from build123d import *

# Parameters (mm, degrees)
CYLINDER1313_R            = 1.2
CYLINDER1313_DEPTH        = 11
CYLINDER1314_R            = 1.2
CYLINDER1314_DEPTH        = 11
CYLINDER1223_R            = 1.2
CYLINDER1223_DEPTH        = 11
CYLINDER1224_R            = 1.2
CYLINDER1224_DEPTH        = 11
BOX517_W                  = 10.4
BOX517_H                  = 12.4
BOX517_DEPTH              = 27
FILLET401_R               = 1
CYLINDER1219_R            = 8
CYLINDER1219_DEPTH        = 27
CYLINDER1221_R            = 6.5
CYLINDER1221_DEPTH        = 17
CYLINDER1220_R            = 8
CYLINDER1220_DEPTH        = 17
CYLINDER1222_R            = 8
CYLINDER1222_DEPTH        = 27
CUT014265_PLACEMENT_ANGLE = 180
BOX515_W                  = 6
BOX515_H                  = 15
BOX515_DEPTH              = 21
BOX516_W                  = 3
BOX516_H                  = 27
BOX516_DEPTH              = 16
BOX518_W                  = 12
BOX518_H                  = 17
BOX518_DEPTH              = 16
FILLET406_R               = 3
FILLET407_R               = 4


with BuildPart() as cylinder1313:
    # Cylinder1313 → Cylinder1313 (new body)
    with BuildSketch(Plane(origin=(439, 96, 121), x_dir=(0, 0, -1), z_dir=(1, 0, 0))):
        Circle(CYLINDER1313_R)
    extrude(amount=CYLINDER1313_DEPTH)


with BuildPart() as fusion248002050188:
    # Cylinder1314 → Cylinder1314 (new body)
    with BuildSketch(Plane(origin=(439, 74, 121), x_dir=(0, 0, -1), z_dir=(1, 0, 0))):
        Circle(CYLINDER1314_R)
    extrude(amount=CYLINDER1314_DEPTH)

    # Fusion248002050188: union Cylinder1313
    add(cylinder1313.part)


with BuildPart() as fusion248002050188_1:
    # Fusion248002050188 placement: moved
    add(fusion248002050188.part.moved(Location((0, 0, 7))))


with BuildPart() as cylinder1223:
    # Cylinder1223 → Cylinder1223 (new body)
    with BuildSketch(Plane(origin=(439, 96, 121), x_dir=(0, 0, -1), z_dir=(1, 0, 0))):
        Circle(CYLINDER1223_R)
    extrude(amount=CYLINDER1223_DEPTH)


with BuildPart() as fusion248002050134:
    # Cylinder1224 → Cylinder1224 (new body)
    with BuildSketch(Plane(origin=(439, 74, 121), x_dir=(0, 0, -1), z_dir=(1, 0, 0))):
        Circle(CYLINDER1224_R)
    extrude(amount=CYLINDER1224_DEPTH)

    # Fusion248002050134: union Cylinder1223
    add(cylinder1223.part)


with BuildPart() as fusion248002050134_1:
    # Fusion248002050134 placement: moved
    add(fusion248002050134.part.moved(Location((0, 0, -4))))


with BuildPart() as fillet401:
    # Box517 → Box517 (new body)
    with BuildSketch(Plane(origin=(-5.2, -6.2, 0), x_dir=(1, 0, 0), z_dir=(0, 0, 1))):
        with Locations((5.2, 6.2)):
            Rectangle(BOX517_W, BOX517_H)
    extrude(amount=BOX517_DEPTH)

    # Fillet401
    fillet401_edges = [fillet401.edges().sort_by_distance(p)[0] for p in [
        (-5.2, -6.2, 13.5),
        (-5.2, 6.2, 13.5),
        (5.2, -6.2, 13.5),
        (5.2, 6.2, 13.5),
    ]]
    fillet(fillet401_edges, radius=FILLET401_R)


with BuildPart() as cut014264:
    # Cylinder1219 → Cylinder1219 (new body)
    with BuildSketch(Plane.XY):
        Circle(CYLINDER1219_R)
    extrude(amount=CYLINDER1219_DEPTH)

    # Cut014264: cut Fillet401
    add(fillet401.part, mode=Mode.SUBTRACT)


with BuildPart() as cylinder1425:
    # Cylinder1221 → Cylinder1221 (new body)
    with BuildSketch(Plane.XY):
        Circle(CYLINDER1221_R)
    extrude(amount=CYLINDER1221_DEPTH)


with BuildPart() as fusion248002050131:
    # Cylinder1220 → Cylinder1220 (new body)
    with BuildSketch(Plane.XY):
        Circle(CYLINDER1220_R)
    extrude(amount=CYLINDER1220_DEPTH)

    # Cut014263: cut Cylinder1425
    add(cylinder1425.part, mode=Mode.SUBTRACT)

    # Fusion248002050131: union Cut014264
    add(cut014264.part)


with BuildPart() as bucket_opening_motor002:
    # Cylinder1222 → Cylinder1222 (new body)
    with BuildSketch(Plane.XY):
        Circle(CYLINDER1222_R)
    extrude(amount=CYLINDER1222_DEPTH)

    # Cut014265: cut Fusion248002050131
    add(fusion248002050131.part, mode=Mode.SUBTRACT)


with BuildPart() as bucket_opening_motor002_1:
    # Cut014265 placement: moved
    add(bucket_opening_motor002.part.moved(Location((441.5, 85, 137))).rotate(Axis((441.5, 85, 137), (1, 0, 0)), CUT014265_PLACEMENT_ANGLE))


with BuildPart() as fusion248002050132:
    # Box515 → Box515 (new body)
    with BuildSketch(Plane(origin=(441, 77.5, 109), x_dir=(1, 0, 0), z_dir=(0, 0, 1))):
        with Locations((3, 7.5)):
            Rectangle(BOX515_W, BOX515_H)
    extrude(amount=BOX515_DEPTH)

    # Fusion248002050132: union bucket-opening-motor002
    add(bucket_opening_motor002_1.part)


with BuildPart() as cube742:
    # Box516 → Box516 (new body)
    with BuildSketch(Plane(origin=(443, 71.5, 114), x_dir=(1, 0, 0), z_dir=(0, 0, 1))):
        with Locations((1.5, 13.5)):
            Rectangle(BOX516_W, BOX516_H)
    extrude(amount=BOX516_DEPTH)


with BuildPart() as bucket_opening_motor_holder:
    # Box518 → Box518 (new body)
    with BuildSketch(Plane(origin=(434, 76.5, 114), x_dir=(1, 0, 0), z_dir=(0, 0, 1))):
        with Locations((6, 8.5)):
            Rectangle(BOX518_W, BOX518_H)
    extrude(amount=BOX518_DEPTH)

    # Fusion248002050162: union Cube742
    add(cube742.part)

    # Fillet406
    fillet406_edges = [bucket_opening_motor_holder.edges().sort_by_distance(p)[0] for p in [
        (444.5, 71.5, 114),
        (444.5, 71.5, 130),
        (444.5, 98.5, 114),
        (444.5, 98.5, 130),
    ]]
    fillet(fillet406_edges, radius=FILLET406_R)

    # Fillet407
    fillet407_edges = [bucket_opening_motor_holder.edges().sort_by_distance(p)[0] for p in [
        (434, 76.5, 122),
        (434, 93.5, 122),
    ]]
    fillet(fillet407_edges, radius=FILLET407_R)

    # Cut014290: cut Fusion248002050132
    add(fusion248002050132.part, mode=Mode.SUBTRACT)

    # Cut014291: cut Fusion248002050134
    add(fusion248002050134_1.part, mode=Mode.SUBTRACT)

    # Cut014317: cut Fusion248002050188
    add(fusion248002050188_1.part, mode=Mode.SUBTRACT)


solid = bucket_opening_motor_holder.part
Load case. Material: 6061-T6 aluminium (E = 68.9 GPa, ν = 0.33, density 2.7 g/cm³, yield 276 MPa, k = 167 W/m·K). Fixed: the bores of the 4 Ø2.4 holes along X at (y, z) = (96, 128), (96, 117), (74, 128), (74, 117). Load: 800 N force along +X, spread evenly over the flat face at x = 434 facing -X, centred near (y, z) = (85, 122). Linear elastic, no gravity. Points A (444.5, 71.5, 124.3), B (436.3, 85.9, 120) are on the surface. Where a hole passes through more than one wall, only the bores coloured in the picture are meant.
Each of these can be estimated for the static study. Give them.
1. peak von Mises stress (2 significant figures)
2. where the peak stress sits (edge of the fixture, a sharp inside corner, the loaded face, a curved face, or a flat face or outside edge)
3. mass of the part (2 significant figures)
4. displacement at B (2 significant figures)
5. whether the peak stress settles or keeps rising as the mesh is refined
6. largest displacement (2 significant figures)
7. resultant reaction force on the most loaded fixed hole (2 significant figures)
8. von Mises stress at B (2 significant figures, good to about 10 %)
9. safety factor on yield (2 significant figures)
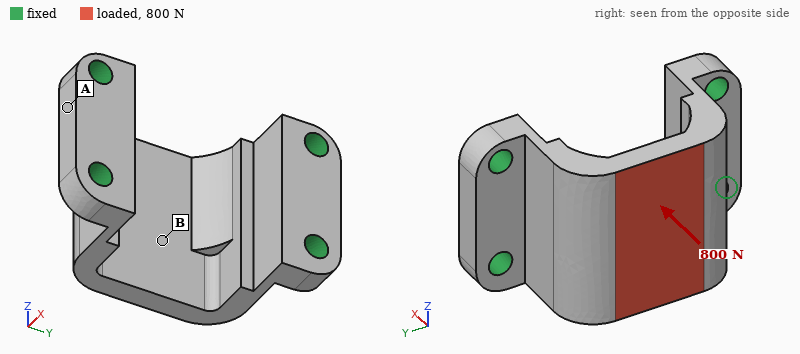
100 MPa
a curved face
4.0 g
14 µm
settles
19 µm
240 N
44 MPa
2.7
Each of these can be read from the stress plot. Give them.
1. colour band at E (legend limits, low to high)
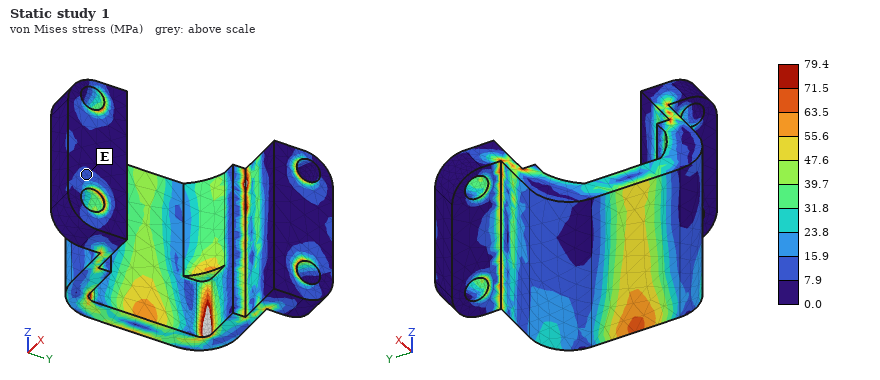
7.9 to 15.9 MPa
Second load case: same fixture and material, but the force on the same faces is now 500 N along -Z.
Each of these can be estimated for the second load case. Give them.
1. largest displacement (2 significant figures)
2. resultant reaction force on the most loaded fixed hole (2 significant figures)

16 µm
270 N
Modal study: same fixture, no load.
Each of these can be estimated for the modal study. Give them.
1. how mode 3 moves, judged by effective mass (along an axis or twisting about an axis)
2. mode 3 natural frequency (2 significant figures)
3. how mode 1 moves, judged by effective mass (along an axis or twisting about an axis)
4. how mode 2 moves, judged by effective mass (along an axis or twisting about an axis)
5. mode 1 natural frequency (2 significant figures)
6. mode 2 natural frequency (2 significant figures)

twisting about X
29 kHz
along Y
along Z
16 kHz
25 kHz
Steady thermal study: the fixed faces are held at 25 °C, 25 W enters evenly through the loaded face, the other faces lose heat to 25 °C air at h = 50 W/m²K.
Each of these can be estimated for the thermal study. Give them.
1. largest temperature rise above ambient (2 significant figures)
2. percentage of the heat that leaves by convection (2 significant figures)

36 K
4.6 %
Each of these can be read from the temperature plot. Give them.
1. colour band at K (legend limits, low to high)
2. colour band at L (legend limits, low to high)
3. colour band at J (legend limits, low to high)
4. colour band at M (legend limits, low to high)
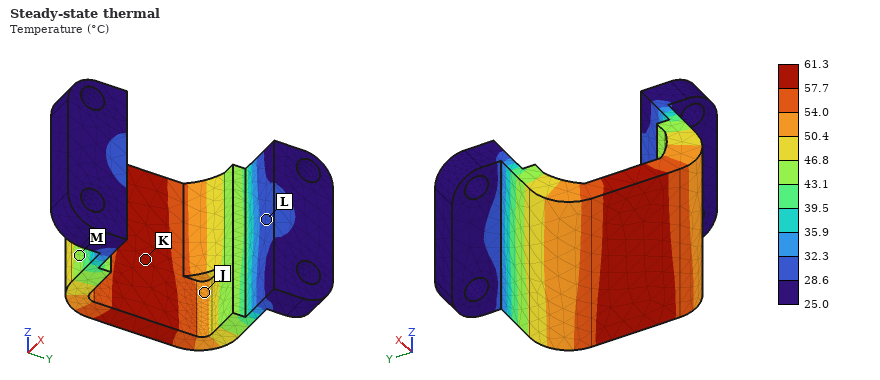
57.7 to 61.3 °C
28.6 to 32.3 °C
50.4 to 54.0 °C
43.1 to 46.8 °C
